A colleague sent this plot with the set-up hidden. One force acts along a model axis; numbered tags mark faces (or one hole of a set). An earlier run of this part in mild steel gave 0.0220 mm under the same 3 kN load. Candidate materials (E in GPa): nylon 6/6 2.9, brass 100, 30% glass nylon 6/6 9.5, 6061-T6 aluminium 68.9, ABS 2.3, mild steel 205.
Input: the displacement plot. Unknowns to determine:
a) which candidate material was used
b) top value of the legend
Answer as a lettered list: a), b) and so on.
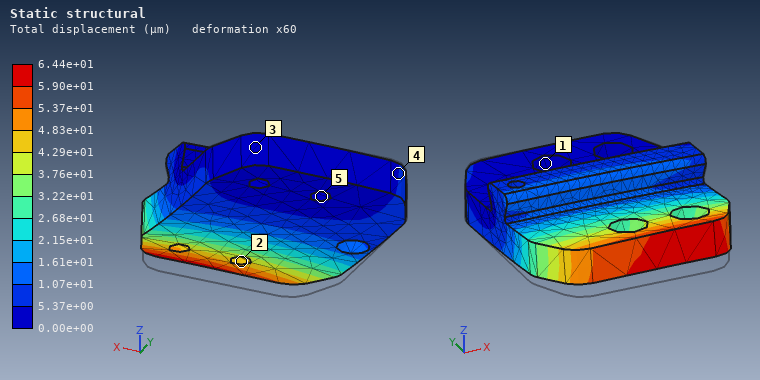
a) 6061-T6 aluminium
b) 6.44e+01 µm
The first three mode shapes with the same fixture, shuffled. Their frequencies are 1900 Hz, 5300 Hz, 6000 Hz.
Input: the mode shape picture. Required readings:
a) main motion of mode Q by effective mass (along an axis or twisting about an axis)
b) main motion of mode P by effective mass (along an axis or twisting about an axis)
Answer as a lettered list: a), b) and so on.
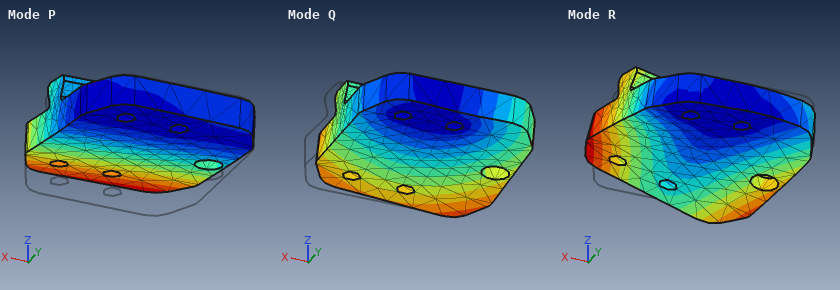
a) along X
b) along Z
